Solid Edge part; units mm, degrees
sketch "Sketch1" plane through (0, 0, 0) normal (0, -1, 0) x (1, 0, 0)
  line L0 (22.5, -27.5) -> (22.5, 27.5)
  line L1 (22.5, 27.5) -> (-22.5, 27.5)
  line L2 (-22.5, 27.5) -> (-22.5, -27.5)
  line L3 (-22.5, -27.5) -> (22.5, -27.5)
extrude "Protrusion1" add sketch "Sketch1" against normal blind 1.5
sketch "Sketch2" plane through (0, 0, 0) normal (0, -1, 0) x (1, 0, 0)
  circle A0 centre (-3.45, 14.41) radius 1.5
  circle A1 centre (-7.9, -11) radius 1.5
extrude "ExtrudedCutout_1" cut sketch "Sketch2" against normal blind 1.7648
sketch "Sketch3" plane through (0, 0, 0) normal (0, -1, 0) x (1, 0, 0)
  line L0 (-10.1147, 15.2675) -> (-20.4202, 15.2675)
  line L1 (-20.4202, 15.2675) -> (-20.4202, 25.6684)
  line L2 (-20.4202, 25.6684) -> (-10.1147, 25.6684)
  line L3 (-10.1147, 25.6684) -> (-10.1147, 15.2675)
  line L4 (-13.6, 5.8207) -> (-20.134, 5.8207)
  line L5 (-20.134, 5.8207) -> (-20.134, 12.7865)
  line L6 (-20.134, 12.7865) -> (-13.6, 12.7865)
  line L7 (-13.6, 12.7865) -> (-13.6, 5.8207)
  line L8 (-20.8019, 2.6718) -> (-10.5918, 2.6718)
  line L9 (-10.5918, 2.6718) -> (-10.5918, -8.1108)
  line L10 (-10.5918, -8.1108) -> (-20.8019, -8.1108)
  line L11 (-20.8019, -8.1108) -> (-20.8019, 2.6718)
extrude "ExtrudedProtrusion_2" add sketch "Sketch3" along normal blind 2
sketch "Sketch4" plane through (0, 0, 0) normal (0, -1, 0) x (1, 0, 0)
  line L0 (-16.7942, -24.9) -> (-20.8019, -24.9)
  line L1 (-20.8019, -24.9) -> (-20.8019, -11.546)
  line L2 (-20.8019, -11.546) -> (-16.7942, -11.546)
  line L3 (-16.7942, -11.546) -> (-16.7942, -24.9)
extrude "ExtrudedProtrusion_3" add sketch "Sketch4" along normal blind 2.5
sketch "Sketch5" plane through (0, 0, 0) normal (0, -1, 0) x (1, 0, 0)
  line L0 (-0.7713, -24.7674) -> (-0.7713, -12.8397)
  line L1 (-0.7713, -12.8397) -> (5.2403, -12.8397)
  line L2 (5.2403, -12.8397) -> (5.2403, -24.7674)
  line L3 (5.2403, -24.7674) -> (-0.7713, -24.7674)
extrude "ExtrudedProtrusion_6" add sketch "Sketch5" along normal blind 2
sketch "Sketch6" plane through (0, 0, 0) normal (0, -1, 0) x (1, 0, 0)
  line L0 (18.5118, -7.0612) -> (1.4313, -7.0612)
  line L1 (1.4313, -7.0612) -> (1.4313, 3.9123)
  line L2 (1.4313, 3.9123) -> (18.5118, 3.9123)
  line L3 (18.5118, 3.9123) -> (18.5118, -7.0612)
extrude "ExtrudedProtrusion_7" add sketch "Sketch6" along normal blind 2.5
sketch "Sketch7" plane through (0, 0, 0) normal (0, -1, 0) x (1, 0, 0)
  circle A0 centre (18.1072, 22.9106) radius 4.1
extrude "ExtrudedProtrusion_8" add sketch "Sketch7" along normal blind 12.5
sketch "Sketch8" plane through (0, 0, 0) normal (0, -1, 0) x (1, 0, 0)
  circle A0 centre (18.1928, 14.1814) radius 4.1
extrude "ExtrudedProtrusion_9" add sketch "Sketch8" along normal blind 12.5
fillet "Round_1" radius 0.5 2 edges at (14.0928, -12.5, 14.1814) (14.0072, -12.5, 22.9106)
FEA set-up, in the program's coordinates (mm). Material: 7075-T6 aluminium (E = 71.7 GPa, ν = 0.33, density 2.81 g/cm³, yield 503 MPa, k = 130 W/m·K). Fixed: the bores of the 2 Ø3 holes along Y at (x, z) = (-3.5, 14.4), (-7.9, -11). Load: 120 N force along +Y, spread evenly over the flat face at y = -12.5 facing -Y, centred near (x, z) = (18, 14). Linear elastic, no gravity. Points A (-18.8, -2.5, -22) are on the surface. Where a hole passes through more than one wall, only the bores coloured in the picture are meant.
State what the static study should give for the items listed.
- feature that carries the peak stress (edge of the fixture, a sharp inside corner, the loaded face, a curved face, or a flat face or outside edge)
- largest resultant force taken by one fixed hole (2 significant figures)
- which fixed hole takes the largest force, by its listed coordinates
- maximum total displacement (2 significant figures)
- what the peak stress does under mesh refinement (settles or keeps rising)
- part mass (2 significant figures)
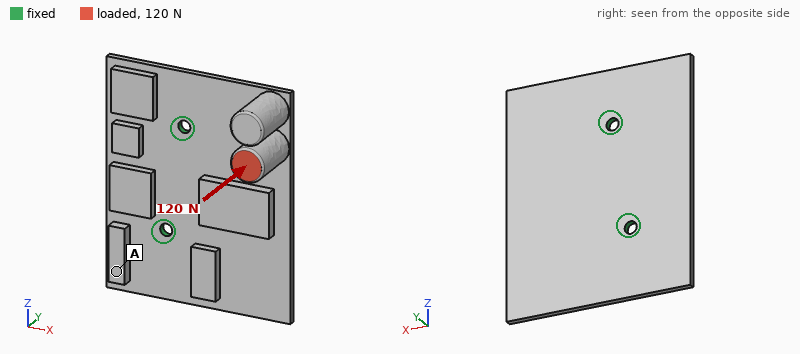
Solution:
edge of the fixture
130 N
(-3.5, 14.4)
0.67 mm
keeps rising
18 g
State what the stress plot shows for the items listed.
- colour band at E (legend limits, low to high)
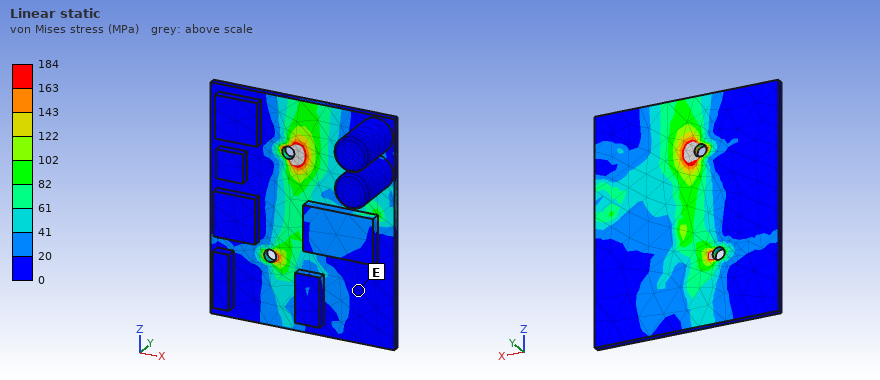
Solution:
0 to 20 MPa
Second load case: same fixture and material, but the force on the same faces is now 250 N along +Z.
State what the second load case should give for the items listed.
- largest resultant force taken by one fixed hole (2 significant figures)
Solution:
270 N
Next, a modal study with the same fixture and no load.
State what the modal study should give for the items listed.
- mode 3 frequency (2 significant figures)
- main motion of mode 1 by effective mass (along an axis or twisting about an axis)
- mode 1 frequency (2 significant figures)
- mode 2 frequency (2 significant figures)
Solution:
2900 Hz
along Y
950 Hz
1700 Hz
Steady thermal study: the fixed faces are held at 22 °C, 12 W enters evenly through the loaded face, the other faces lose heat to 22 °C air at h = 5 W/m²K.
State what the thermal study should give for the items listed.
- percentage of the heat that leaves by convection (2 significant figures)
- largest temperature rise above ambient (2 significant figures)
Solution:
4.1 %
66 K
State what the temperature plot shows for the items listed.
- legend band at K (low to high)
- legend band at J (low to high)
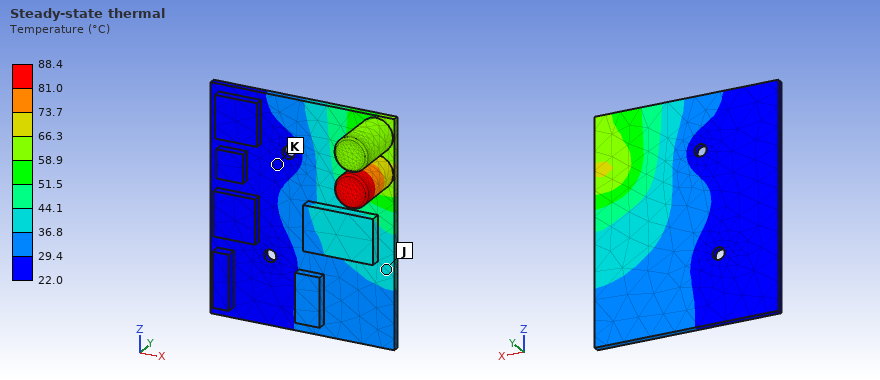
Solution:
22.0 to 29.4 °C
36.8 to 44.1 °C
